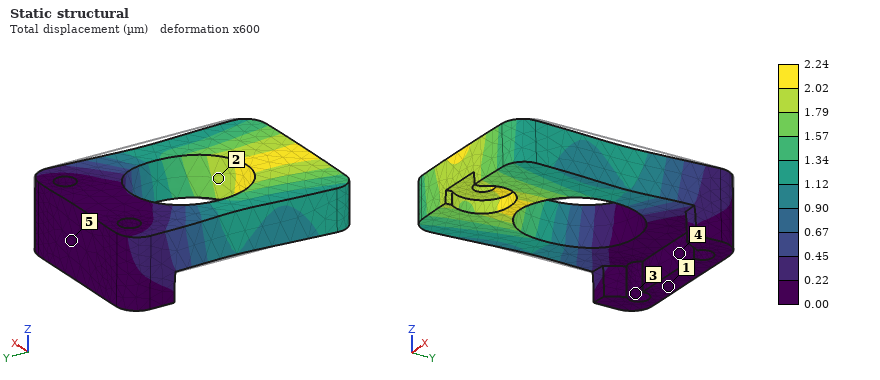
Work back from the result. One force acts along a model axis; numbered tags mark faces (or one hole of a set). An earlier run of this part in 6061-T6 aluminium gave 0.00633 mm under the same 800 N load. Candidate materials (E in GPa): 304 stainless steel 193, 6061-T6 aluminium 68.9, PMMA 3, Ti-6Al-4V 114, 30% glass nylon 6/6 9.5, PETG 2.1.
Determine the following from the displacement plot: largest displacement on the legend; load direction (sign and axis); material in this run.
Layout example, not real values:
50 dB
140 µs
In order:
2.24 µm
-Y
304 stainless steel
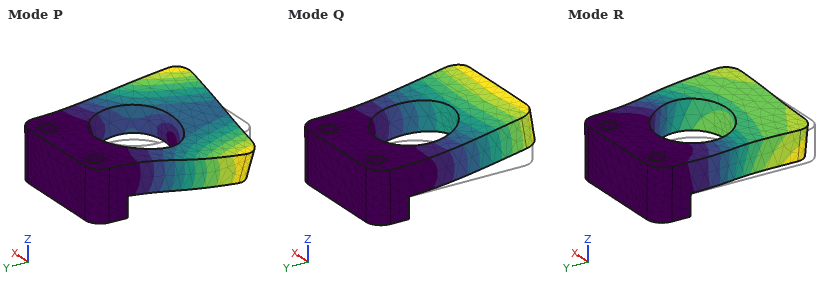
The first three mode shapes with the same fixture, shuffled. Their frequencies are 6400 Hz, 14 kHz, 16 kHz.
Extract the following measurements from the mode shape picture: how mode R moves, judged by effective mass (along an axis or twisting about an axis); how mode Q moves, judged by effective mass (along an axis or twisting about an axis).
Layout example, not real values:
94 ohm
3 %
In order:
along X
along Z
